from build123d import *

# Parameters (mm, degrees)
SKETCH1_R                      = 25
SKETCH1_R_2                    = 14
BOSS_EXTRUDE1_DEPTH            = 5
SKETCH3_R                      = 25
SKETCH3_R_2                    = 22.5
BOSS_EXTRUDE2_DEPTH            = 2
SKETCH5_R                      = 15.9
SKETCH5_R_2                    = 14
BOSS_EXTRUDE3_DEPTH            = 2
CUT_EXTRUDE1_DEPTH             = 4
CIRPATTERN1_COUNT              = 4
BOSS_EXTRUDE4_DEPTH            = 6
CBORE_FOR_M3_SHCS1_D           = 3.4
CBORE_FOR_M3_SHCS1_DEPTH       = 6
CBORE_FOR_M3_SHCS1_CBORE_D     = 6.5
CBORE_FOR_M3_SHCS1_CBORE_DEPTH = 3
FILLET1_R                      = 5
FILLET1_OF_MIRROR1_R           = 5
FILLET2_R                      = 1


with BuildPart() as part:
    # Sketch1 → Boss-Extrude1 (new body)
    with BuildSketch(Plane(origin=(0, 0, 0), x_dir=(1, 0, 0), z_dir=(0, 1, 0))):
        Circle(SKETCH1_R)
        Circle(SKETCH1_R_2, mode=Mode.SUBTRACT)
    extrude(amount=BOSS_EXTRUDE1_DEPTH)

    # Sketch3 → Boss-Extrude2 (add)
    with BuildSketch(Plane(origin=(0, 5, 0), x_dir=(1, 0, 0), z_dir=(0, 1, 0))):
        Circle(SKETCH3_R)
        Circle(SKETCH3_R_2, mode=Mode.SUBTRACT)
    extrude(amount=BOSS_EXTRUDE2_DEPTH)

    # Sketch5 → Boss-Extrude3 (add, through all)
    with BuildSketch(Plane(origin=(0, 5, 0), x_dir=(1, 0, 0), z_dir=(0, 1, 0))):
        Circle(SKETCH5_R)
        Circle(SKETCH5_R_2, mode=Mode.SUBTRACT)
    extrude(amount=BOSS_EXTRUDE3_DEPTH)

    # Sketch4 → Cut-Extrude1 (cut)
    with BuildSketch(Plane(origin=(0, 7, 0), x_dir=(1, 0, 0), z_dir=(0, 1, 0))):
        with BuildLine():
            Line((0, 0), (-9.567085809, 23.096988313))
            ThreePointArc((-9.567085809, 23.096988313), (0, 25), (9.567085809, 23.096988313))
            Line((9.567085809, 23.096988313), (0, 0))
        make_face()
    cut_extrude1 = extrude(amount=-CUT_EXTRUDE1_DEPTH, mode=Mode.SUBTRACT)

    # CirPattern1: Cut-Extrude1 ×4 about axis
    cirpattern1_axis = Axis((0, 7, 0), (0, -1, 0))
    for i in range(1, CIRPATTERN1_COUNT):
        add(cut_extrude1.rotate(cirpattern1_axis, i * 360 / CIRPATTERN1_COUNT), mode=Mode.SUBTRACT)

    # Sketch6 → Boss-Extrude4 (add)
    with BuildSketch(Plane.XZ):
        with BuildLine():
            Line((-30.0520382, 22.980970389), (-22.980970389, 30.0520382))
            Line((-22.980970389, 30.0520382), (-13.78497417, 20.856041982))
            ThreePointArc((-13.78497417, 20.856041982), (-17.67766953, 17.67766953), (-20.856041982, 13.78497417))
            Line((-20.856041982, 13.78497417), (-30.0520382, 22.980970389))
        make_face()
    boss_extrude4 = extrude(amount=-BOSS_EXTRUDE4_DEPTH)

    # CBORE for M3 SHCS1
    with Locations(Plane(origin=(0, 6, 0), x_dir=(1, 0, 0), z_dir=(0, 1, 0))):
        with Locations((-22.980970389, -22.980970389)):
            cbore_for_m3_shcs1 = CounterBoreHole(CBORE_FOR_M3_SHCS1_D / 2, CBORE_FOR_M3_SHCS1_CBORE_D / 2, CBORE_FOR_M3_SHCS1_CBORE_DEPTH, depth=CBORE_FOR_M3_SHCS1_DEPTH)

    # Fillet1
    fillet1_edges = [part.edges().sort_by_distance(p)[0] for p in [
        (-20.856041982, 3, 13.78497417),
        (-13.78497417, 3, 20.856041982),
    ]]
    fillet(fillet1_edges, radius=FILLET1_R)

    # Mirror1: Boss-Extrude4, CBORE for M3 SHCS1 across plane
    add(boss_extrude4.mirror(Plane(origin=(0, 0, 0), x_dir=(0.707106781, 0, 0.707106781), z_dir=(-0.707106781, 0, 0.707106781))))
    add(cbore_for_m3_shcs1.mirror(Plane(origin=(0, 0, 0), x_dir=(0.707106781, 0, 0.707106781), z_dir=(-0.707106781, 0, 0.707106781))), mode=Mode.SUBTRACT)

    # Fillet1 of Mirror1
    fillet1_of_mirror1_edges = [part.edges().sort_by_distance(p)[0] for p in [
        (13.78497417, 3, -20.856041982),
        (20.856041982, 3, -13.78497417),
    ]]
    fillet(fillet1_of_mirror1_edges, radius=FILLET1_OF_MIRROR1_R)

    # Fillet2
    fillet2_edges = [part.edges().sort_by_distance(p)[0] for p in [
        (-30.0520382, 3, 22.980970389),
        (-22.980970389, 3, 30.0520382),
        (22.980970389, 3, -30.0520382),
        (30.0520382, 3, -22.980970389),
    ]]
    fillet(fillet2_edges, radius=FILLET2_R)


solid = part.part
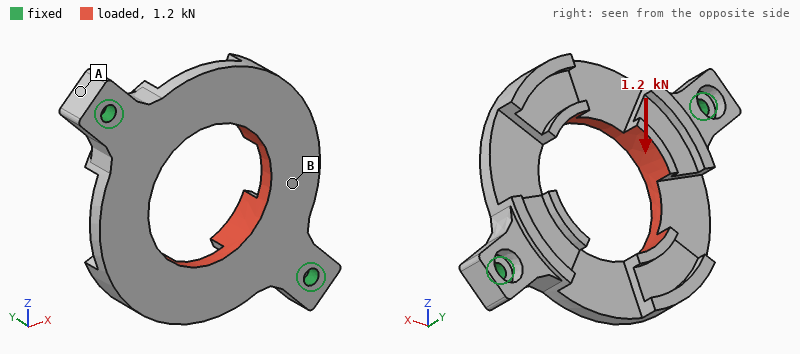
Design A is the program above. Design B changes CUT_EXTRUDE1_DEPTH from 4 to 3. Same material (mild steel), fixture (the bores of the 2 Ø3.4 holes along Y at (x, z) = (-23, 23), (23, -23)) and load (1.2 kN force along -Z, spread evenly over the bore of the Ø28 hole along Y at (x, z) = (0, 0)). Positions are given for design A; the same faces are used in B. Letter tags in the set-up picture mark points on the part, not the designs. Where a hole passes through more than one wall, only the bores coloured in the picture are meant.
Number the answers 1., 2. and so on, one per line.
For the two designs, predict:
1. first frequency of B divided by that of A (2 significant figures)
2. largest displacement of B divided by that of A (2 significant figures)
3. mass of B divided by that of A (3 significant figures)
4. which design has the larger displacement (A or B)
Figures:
1. 1.1
2. 0.65
3. 1.09
4. A
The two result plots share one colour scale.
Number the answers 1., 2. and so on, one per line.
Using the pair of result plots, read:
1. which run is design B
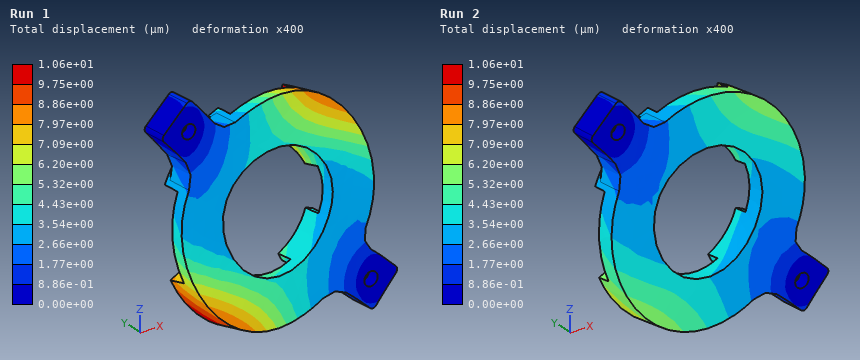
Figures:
1. Run 2
